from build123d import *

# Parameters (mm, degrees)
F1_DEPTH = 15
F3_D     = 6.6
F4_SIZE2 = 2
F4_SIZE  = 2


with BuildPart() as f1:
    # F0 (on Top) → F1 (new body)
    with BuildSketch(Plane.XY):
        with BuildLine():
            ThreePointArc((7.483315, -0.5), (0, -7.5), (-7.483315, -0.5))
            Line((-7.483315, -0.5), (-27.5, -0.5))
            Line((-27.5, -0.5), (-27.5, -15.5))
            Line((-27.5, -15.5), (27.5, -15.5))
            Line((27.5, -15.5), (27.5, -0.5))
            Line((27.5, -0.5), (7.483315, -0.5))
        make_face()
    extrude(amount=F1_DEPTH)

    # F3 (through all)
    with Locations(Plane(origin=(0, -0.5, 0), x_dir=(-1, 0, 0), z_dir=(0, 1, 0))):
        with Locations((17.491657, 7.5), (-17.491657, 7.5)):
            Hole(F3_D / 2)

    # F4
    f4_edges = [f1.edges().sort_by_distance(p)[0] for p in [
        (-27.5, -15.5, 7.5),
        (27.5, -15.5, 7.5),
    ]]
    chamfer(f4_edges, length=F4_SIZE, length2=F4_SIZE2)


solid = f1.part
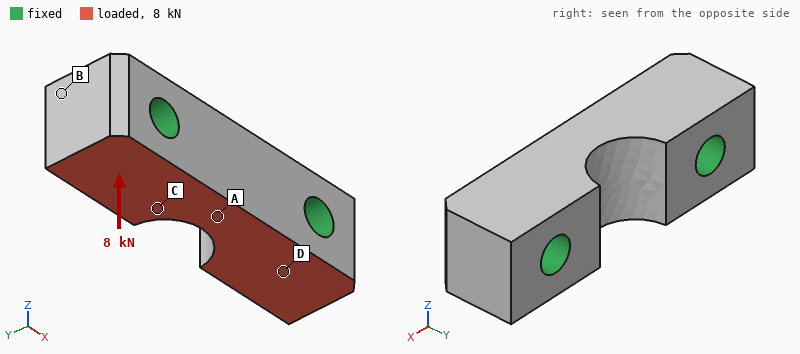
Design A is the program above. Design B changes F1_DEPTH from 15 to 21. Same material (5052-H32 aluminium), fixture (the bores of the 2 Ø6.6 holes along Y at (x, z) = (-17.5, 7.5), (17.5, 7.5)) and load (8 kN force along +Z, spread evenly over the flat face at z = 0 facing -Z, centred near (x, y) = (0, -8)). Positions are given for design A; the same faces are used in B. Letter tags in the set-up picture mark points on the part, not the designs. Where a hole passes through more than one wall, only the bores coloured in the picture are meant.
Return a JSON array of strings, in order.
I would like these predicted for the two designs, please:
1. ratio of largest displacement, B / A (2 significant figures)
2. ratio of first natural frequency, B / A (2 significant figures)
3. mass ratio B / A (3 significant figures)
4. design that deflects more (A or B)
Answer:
["0.77", "0.86", "1.44", "A"]
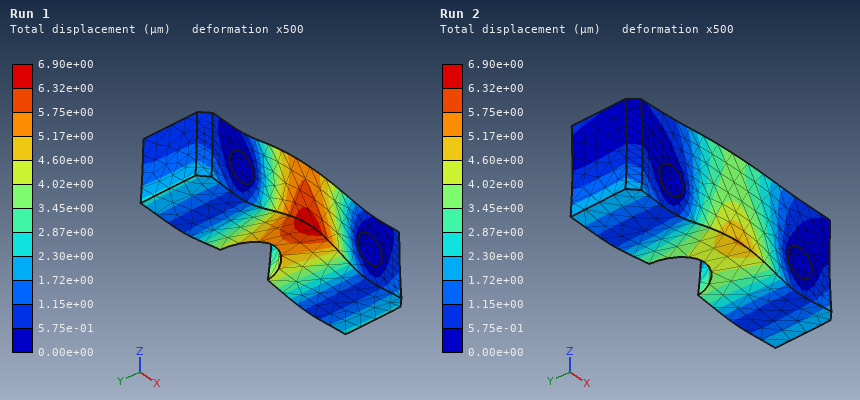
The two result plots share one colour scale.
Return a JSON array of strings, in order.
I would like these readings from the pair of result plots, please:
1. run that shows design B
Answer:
["Run 2"]
